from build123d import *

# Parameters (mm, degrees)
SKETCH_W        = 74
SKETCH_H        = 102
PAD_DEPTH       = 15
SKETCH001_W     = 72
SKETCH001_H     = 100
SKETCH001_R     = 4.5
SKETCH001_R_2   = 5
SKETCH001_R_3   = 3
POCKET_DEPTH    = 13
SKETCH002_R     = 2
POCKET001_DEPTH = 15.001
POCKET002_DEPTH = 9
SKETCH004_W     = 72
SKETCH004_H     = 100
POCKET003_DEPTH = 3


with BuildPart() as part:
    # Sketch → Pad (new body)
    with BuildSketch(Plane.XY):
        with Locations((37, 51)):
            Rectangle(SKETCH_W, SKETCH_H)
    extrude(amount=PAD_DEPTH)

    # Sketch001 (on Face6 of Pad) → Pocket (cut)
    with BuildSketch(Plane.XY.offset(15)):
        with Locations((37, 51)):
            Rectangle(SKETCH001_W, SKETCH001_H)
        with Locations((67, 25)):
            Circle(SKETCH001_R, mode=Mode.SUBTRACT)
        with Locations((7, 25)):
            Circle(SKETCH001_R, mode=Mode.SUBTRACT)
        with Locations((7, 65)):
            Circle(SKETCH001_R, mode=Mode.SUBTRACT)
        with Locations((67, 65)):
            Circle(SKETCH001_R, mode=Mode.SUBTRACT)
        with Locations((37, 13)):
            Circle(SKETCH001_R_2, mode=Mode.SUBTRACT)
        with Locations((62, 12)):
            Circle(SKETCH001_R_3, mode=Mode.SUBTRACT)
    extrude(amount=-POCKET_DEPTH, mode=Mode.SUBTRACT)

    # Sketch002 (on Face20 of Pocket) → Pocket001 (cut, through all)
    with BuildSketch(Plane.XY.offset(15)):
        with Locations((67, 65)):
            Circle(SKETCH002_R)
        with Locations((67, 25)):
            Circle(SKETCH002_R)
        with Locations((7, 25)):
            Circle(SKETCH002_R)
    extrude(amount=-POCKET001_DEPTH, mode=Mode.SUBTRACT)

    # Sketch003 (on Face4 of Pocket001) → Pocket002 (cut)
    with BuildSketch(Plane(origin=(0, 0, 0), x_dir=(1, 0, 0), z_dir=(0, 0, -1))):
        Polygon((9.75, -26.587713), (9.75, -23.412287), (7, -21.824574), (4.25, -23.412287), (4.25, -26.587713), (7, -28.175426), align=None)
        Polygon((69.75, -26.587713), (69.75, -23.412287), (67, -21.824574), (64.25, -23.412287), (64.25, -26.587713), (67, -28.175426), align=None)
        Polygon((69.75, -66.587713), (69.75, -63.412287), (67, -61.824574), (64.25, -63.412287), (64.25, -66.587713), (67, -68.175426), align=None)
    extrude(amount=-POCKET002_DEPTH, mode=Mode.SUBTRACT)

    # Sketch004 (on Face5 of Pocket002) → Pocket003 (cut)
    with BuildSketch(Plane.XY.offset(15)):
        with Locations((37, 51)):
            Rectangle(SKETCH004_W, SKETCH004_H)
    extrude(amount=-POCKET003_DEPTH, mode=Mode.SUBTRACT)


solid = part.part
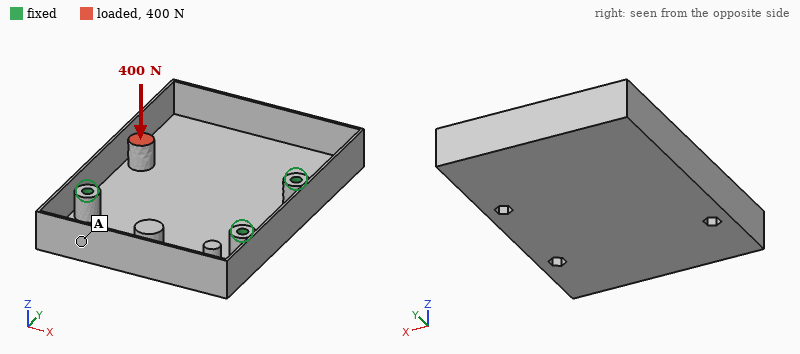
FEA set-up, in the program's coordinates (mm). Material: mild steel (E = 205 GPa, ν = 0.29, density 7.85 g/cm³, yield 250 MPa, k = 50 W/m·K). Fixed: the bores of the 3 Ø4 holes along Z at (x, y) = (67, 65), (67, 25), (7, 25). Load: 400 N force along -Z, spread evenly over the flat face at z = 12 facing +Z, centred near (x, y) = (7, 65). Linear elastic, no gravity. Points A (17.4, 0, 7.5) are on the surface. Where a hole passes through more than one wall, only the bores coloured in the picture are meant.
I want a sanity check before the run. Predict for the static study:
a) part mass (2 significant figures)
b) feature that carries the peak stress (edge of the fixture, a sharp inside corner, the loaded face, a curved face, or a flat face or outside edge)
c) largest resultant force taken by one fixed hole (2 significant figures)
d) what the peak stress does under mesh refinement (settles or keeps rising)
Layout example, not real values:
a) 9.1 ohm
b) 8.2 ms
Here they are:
a) 180 g
b) edge of the fixture
c) 440 N
d) keeps rising
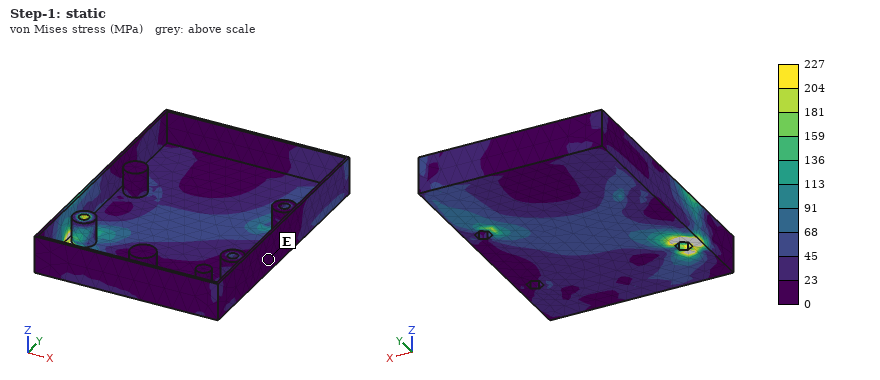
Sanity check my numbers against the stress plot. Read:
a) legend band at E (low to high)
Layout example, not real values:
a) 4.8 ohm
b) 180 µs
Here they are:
a) 0 to 23 MPa
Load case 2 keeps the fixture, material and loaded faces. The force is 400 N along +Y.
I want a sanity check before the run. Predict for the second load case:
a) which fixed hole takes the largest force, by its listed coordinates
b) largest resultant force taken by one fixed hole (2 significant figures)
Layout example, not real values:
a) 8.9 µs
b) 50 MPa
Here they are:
a) (7, 25)
b) 390 N
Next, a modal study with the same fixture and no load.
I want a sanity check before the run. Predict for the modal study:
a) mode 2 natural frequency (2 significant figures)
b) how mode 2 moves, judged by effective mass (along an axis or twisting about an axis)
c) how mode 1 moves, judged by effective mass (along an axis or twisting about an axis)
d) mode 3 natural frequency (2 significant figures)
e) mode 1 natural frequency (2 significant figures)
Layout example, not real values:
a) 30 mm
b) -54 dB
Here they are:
a) 2400 Hz
b) along Z
c) along Z
d) 2800 Hz
e) 660 Hz
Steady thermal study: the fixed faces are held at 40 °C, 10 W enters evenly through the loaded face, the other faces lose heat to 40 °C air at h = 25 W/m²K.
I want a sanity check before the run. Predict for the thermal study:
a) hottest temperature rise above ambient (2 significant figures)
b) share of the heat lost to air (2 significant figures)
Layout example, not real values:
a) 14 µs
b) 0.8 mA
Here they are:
a) 83 K
b) 75 %
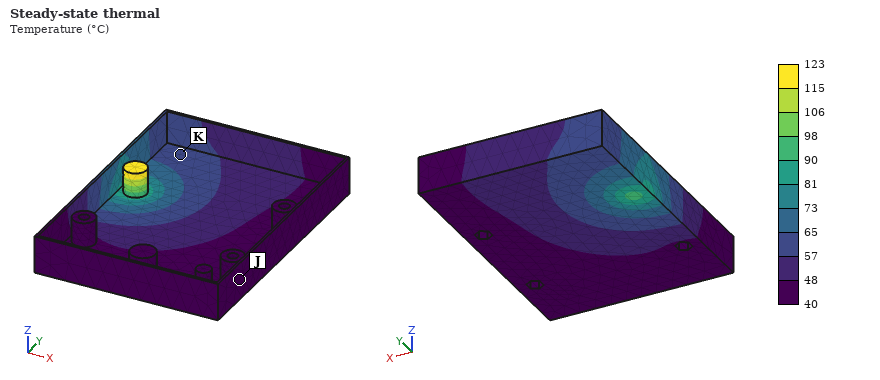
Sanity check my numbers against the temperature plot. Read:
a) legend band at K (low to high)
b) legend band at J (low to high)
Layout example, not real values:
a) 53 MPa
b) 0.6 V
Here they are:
a) 57 to 65 °C
b) 40 to 48 °C
